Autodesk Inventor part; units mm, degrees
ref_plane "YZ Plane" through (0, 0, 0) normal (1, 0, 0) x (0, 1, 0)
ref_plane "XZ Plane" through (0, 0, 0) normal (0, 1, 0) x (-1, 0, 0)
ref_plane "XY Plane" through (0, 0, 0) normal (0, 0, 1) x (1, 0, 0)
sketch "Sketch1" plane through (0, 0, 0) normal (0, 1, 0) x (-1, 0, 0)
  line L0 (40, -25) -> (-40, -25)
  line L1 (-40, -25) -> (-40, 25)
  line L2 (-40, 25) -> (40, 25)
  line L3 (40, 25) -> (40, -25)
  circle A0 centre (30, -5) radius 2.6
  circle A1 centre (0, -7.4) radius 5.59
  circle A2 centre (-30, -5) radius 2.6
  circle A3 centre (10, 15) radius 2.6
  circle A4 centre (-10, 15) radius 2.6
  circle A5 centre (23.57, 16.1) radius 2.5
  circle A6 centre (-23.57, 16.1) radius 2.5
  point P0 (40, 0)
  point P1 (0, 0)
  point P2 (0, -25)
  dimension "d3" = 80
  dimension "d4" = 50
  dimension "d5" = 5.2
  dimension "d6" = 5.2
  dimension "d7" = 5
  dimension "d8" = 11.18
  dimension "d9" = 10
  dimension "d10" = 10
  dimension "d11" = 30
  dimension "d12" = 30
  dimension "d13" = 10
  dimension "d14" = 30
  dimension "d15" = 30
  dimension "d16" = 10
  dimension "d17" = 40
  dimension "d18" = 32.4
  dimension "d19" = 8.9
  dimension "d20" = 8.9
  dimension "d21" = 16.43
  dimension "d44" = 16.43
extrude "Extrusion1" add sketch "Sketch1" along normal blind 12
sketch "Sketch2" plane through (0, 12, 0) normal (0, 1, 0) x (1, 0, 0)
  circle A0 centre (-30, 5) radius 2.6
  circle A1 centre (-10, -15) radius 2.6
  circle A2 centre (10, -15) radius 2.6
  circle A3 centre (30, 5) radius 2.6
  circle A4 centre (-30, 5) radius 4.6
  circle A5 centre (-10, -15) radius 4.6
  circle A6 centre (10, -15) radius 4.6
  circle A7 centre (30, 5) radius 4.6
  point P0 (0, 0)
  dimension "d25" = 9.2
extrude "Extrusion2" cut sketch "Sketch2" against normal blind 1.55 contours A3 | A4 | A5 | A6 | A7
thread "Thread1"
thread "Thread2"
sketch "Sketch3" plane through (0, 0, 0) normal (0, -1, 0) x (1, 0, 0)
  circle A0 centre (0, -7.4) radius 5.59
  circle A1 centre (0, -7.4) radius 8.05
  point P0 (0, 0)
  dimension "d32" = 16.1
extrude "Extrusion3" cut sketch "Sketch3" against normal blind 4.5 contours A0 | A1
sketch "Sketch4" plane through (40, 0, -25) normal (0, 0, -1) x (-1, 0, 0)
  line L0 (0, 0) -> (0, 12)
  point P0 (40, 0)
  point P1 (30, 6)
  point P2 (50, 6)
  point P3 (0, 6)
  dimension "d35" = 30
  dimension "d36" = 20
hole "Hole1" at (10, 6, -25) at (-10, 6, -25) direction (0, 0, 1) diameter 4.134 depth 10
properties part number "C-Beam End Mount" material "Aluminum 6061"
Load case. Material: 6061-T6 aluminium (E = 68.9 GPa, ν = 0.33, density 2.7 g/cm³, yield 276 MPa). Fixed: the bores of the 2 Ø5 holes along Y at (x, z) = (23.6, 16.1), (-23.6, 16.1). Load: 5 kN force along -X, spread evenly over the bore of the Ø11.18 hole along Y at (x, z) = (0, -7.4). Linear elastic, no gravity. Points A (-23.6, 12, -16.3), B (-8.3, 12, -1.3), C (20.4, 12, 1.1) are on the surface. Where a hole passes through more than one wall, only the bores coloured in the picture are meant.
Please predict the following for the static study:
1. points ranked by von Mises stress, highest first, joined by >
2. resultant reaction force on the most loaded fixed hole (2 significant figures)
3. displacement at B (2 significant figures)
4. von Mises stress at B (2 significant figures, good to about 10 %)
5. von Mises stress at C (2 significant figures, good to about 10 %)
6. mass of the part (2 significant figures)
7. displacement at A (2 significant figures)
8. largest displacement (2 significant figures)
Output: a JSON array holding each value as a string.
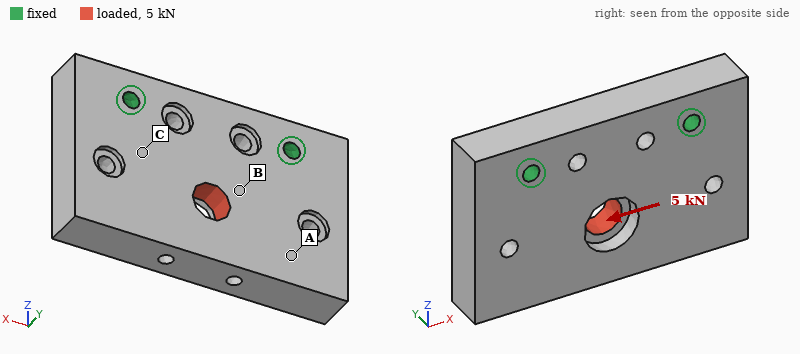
["B > C > A", "3.4 kN", "8.0 µm", "20 MPa", "12 MPa", "120 g", "13 µm", "16 µm"]
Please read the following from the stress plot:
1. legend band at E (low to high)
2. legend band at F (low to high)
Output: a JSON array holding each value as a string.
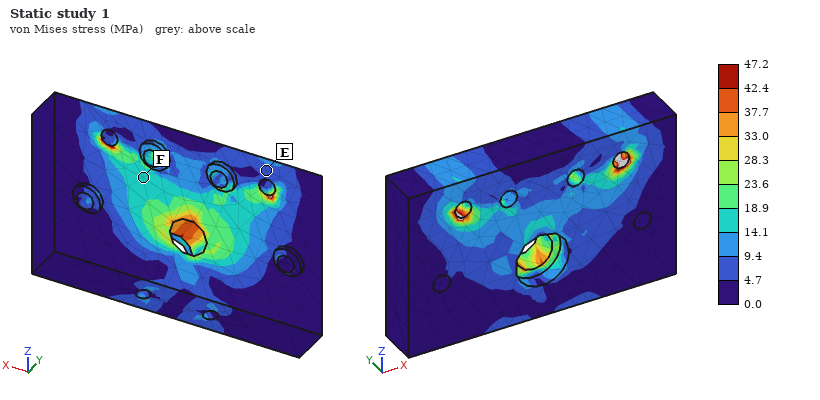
["4.7 to 9.4 MPa", "14.1 to 18.9 MPa"]
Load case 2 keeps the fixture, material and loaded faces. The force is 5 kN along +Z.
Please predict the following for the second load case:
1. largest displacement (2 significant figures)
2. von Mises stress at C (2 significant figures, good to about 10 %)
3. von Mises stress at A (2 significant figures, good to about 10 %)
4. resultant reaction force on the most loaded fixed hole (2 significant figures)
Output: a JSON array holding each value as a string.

["20 µm", "14 MPa", "3.8 MPa", "2.7 kN"]
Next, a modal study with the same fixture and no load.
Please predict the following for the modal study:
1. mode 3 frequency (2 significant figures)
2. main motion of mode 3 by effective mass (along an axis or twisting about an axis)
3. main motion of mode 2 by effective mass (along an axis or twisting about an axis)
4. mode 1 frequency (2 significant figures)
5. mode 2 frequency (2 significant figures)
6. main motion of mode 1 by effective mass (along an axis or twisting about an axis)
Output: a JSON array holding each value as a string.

["11 kHz", "along X", "twisting about Z", "4400 Hz", "6800 Hz", "along Y"]
